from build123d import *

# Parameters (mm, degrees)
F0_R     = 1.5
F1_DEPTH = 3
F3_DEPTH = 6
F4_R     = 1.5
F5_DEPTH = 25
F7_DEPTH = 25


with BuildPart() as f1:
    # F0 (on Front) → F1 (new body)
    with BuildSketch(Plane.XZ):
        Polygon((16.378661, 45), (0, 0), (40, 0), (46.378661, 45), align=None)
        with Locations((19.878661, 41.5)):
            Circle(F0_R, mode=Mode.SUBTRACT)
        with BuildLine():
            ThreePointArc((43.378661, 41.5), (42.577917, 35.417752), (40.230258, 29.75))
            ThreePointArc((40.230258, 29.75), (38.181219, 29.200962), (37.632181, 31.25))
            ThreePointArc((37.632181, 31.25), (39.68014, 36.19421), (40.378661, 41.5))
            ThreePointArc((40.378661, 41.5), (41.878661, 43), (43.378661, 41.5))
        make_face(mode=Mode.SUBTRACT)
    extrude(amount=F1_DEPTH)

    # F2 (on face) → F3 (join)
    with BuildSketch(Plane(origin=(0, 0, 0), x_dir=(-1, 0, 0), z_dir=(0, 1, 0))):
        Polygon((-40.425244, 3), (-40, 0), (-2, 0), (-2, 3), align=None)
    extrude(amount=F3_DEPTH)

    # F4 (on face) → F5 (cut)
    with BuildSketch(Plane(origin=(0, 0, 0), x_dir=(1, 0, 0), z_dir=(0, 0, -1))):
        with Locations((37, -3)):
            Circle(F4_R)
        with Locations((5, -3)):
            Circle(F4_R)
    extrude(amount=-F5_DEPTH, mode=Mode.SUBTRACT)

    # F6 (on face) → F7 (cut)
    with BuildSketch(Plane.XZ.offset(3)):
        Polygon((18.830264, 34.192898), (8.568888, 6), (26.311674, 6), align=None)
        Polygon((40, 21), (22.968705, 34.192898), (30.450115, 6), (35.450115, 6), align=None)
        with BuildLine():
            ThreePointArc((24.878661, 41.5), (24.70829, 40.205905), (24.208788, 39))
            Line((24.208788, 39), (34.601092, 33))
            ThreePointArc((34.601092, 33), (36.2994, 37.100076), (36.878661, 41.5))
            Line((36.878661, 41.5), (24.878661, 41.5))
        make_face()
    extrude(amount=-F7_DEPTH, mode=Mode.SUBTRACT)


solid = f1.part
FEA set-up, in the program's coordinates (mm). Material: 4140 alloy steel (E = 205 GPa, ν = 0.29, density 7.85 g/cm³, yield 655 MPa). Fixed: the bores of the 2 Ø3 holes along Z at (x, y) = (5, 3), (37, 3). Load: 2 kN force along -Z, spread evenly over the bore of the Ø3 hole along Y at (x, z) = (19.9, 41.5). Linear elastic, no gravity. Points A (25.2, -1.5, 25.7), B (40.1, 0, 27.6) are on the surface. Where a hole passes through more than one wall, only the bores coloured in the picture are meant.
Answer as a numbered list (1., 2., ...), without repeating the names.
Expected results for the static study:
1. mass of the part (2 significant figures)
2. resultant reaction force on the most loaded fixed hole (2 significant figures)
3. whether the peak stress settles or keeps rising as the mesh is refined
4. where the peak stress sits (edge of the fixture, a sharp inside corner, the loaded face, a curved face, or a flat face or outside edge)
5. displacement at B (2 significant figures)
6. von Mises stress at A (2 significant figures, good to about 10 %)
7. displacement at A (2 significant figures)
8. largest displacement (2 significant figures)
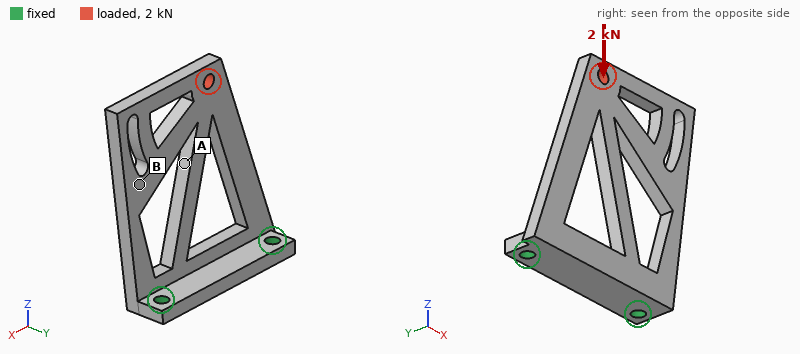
1. 28 g
2. 1.1 kN
3. keeps rising
4. edge of the fixture
5. 54 µm
6. 82 MPa
7. 54 µm
8. 94 µm
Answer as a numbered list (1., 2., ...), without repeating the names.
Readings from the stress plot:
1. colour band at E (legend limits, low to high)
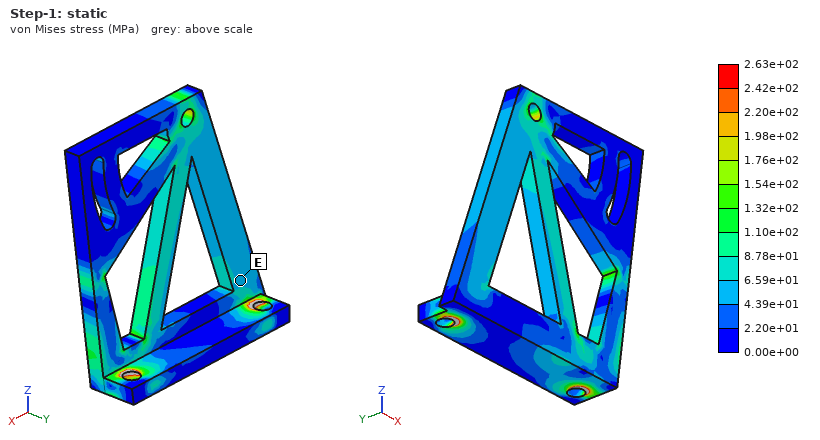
1. 4.39e+01 to 6.59e+01 MPa
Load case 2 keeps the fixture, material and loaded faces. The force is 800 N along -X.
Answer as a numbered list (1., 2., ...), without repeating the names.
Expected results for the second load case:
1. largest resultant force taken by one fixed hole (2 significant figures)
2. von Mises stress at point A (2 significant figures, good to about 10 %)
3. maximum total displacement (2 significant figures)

1. 1.1 kN
2. 43 MPa
3. 76 µm
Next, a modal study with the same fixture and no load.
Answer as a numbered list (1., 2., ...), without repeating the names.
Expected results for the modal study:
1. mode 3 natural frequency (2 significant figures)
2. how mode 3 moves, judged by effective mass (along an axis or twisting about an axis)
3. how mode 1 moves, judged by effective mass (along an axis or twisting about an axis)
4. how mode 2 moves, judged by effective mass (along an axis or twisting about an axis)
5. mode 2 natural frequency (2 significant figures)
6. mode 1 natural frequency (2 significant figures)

1. 5500 Hz
2. along X
3. along Y
4. twisting about Z
5. 2900 Hz
6. 980 Hz
